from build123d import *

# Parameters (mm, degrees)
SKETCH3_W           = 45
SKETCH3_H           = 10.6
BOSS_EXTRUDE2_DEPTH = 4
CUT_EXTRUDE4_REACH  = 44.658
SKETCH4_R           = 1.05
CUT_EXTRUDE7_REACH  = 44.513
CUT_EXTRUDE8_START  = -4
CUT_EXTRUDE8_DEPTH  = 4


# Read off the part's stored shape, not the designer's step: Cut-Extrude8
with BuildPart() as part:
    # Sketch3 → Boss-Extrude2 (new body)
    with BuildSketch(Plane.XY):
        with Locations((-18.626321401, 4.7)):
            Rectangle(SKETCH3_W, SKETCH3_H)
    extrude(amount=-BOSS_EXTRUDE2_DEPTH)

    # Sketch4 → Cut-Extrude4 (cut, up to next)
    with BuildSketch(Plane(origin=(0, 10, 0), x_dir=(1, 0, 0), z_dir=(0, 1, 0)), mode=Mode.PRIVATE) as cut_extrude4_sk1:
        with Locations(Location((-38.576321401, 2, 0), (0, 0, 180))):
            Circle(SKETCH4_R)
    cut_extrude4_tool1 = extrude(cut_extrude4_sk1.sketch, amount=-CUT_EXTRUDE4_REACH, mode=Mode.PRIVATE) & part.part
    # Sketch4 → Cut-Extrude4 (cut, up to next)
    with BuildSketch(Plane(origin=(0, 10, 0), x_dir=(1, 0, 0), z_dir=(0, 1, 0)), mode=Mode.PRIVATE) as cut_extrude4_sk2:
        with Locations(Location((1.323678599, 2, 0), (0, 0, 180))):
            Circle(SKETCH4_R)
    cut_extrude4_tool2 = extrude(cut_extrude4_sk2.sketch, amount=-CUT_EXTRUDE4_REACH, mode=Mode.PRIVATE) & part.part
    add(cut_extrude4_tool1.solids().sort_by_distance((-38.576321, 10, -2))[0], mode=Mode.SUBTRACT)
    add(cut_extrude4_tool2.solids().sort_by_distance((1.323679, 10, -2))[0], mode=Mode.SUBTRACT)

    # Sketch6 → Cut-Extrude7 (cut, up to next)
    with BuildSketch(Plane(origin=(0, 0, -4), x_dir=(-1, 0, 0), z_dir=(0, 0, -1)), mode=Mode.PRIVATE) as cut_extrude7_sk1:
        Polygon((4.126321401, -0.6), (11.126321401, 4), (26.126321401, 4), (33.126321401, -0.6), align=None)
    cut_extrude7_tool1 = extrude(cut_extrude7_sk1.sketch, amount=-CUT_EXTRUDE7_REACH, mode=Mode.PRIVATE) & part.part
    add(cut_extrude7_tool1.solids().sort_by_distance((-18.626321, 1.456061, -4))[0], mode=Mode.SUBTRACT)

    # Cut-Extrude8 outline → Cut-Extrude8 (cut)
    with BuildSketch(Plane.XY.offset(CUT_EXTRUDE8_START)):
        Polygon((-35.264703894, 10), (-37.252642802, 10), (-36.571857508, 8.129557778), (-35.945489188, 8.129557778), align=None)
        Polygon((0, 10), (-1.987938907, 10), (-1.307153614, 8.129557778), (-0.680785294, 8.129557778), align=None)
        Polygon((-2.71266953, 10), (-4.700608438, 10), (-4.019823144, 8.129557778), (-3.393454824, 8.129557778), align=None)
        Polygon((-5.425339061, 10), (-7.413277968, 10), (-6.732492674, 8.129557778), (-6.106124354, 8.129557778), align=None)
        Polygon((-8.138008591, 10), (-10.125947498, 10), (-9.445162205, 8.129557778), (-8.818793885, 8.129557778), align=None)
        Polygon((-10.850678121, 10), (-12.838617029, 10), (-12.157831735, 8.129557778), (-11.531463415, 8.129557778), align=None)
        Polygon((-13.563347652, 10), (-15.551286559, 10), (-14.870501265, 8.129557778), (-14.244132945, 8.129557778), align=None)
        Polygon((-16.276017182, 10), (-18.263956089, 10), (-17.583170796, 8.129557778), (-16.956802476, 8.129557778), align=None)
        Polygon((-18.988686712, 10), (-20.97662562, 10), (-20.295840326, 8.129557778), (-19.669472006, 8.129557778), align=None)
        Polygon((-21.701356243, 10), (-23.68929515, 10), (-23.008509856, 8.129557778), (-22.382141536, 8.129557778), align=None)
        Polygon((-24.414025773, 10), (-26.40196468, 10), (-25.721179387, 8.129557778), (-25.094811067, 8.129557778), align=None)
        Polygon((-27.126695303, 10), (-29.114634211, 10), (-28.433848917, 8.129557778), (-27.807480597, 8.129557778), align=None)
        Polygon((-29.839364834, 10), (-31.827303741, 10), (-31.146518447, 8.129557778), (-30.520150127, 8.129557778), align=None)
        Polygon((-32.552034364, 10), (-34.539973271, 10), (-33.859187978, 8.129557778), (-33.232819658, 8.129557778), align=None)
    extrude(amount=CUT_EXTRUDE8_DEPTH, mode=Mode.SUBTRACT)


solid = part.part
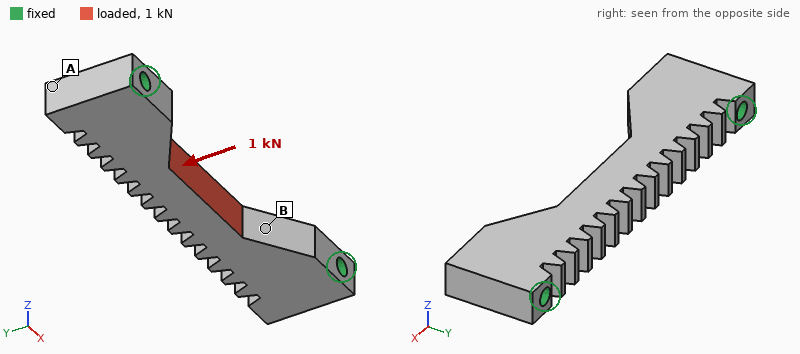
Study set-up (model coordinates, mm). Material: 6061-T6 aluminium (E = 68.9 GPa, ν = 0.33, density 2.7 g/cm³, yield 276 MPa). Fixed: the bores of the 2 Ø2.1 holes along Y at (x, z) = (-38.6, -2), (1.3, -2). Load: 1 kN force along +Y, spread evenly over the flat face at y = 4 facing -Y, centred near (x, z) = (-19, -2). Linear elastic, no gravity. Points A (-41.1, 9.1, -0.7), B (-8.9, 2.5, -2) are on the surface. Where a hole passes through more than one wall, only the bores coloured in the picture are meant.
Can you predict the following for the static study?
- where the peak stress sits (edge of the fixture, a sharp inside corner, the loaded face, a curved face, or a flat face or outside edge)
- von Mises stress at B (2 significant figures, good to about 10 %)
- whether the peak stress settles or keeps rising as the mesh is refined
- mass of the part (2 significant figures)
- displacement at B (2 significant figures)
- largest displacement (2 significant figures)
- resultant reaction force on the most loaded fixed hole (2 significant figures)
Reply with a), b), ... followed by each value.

a) edge of the fixture
b) 99 MPa
c) keeps rising
d) 3.5 g
e) 19 µm
f) 50 µm
g) 620 N
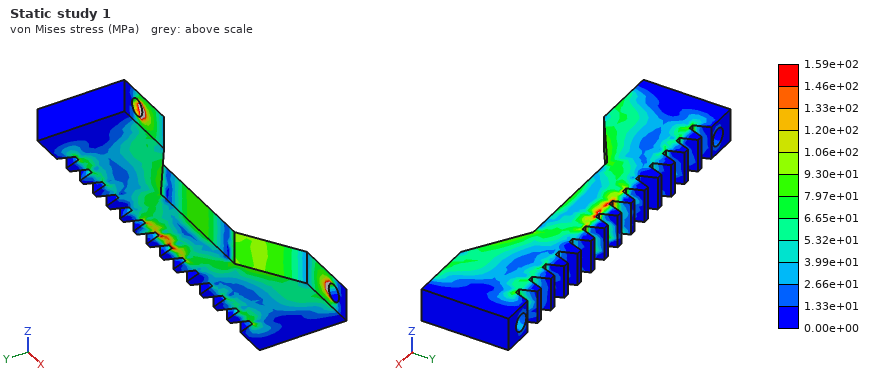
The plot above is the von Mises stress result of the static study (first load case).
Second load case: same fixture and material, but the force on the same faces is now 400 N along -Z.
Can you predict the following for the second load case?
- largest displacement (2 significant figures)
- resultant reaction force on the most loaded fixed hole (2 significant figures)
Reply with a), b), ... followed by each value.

a) 62 µm
b) 200 N
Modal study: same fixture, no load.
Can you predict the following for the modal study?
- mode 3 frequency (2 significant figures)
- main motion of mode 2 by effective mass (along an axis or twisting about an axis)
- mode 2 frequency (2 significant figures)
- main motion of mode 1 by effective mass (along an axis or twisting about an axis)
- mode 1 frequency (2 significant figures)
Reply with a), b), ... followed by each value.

a) 30 kHz
b) along Y
c) 24 kHz
d) along Z
e) 13 kHz
